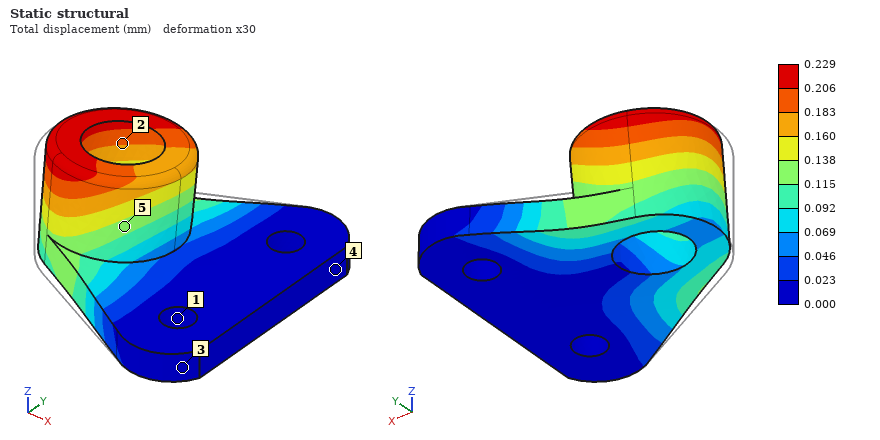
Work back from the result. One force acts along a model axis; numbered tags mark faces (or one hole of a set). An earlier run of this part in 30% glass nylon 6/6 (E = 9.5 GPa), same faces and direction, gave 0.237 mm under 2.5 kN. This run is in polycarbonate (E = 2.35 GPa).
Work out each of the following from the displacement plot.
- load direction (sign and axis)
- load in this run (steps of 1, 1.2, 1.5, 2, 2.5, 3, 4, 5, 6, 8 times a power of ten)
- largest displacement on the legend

+Y
600 N
0.229 mm
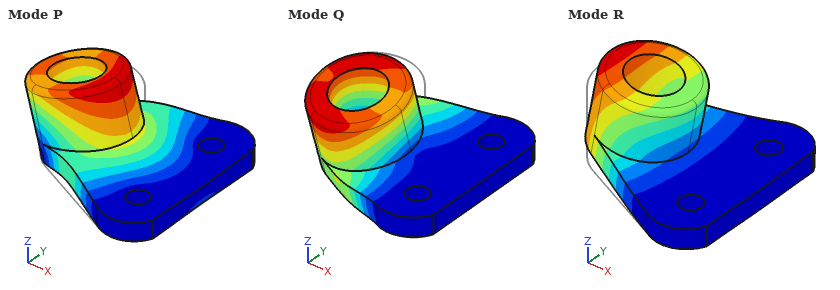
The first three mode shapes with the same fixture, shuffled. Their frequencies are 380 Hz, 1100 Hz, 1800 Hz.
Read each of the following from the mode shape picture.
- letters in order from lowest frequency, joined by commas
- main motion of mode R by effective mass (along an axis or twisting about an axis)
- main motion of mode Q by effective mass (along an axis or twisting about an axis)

R, Q, P
along Z
along Y
